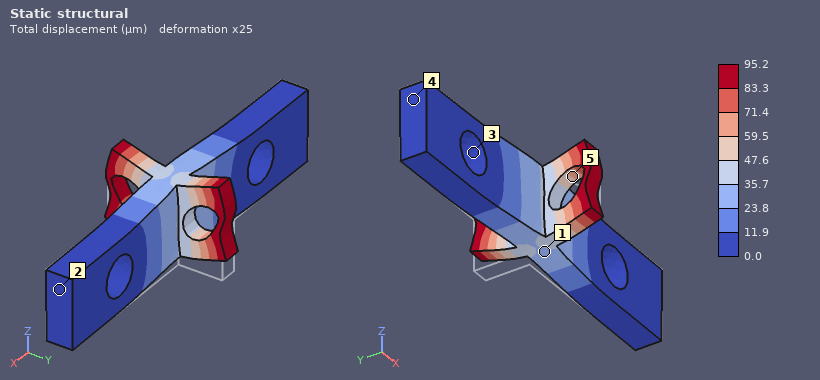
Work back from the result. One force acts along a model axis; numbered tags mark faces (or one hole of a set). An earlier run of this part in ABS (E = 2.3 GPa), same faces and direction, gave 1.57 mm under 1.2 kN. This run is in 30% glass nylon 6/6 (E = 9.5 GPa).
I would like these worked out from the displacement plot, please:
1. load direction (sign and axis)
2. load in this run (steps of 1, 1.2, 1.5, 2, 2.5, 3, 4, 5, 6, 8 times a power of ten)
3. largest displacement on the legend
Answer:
+Z
300 N
95.2 µm
